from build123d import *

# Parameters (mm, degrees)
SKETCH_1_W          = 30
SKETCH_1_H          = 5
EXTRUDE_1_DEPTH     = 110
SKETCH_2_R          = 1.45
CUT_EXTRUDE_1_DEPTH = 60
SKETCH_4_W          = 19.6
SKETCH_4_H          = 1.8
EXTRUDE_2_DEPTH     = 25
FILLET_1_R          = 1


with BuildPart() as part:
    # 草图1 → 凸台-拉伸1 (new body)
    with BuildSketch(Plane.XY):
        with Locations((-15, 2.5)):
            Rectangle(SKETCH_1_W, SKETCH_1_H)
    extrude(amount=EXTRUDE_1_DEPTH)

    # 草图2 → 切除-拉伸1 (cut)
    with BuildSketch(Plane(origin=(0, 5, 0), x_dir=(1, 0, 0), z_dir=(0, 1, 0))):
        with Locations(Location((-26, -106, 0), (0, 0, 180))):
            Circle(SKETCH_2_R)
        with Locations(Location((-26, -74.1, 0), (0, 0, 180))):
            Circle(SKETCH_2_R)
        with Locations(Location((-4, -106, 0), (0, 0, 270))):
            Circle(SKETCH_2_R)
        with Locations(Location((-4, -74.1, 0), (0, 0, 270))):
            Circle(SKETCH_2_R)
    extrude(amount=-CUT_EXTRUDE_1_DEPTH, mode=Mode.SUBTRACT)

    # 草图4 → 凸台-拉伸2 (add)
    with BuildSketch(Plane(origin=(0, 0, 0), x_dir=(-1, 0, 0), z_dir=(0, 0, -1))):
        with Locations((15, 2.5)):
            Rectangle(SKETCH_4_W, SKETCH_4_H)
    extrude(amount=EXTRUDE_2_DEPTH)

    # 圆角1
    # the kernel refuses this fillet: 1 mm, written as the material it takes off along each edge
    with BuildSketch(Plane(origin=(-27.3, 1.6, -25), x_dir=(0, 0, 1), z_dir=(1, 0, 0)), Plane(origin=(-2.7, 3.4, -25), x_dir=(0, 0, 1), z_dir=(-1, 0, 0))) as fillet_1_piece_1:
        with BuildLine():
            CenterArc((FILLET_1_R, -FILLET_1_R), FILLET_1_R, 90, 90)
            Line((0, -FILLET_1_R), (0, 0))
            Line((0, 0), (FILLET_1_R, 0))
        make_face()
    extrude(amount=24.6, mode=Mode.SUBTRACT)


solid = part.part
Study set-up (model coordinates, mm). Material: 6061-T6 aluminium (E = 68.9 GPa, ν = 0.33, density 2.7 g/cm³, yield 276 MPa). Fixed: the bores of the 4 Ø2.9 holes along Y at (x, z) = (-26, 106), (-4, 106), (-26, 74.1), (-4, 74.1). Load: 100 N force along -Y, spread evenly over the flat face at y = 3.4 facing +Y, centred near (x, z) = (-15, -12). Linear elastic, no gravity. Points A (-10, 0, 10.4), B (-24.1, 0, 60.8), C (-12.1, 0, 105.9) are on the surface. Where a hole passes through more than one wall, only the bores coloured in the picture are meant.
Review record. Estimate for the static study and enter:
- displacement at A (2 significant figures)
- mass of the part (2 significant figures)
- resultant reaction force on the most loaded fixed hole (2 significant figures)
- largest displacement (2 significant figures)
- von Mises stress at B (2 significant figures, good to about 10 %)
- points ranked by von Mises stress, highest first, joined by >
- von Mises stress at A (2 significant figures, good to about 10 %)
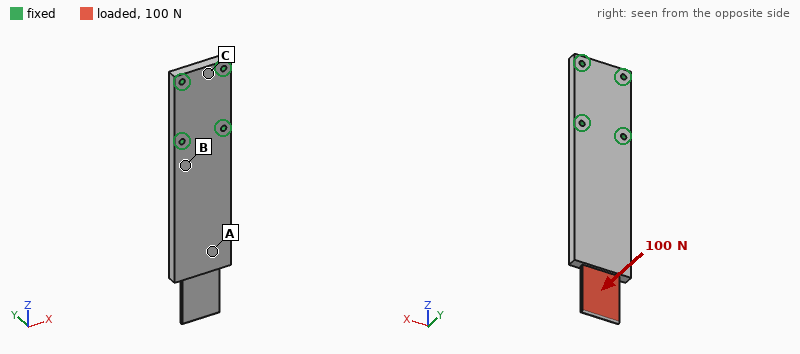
0.63 mm
47 g
85 N
1.5 mm
57 MPa
B > A > C
20 MPa
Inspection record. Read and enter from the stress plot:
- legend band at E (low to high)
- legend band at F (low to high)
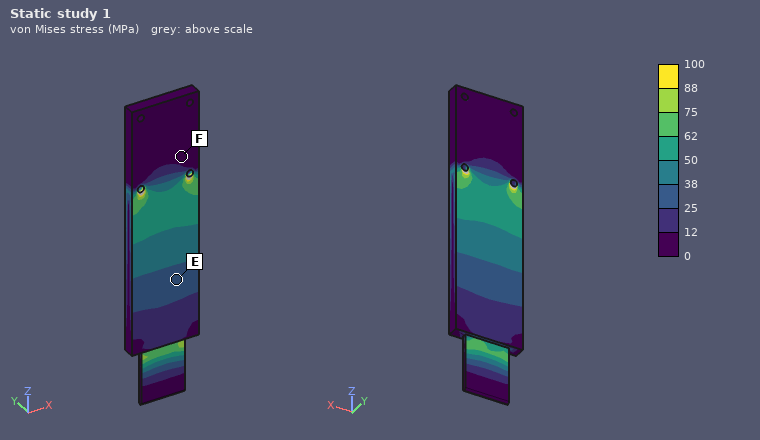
25 to 38 MPa
0 to 12 MPa
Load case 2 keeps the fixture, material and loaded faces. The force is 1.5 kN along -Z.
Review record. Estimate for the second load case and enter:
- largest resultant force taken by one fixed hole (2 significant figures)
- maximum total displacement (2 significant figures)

680 N
0.71 mm
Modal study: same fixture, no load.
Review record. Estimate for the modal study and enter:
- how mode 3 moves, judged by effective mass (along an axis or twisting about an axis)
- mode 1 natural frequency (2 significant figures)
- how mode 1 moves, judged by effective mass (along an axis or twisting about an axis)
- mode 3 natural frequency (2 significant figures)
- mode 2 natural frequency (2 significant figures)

along X
590 Hz
along Y
3300 Hz
2300 Hz
